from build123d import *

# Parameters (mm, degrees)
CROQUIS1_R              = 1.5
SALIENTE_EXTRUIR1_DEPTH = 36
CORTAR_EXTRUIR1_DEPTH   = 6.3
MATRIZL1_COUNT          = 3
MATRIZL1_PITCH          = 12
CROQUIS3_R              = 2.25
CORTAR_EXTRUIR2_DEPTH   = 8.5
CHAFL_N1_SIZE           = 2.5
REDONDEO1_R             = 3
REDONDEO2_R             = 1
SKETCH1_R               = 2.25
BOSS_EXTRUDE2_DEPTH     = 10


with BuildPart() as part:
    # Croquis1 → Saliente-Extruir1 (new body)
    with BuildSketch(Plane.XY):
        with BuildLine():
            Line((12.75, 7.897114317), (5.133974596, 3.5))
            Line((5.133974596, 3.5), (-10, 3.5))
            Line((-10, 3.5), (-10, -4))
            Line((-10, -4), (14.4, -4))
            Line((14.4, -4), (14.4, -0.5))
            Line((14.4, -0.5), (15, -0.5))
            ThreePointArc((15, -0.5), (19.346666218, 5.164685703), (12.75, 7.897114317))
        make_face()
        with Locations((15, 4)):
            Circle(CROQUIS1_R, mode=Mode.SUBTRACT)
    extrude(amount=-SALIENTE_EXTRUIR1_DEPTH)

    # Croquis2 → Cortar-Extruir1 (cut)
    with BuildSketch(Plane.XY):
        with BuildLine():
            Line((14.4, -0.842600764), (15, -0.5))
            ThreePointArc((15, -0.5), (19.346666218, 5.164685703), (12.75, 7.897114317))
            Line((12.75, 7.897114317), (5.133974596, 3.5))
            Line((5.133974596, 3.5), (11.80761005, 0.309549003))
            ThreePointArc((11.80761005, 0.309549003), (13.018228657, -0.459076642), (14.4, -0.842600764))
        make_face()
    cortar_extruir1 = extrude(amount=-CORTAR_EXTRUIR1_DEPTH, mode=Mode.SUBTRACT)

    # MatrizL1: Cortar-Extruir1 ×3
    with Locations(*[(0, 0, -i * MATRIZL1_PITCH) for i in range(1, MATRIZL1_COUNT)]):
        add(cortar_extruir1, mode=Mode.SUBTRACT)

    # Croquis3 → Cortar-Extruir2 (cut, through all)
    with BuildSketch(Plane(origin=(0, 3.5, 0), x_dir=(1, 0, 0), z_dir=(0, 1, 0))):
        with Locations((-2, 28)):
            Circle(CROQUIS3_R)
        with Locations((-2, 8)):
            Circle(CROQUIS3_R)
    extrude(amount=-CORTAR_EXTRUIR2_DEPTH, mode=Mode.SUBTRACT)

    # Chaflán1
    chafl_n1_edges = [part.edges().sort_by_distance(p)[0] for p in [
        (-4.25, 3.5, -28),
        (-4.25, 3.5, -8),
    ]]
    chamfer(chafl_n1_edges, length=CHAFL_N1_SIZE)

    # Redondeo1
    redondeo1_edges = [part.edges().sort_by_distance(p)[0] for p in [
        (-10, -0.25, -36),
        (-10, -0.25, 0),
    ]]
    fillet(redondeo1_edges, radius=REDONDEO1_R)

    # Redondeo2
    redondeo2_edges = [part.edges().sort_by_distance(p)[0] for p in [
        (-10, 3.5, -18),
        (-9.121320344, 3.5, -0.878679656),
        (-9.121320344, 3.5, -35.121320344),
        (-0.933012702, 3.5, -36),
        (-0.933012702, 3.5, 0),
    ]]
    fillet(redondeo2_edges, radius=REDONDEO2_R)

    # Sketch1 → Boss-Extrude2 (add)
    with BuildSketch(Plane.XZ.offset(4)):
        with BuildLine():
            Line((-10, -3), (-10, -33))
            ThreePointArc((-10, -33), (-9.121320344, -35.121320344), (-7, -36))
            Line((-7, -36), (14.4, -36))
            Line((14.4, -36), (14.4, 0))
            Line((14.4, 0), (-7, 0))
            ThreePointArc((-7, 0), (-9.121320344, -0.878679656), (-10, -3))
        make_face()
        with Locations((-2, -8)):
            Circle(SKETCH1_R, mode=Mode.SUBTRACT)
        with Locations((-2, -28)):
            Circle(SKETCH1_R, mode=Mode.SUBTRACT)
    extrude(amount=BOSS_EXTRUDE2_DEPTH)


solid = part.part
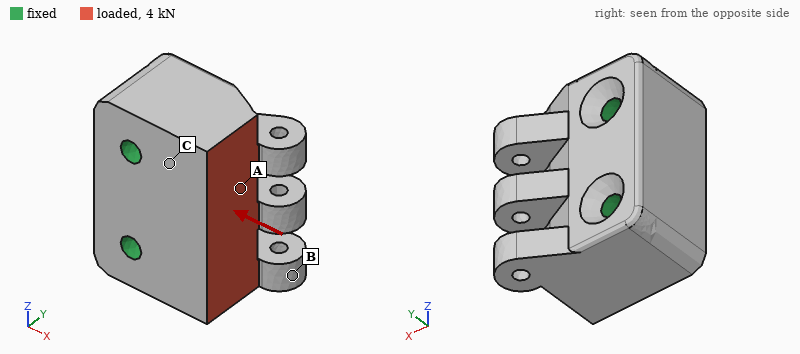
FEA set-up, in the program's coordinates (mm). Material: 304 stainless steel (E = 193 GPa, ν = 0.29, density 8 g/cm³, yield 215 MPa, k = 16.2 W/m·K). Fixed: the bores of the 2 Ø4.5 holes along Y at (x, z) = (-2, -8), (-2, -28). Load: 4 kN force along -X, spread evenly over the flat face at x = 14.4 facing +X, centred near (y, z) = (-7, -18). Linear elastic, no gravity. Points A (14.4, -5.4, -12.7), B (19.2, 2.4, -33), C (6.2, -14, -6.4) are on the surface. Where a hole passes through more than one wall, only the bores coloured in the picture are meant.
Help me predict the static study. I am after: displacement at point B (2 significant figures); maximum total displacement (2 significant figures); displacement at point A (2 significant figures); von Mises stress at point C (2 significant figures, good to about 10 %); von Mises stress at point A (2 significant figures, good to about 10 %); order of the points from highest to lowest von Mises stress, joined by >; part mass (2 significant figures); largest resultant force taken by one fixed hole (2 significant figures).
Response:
0.67 µm
1.1 µm
0.77 µm
11 MPa
7.0 MPa
C > A > B
120 g
2.0 kN
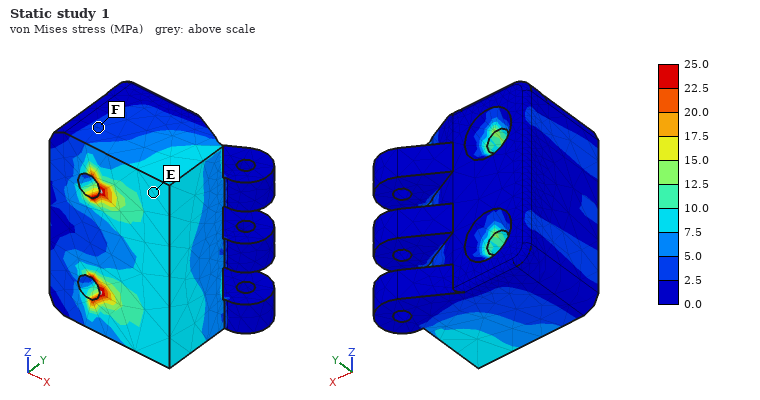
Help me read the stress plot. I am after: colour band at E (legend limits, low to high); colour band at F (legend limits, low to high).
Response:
7.5 to 10.0 MPa
2.5 to 5.0 MPa
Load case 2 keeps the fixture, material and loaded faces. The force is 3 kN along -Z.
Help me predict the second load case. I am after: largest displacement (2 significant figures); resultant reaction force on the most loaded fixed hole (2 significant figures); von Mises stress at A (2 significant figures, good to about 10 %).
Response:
2.9 µm
2.5 kN
13 MPa
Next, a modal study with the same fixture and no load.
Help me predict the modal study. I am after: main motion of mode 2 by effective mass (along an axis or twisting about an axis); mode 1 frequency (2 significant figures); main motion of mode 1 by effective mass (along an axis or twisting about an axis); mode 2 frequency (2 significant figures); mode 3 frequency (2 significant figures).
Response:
along Z
23 kHz
along Y
26 kHz
30 kHz
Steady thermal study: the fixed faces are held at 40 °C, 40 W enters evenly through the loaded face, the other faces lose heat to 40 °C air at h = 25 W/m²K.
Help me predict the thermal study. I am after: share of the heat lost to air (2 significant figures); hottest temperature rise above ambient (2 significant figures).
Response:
6.5 %
74 K
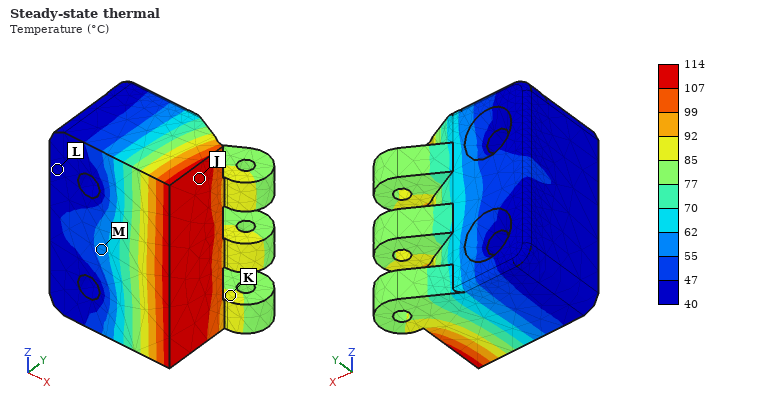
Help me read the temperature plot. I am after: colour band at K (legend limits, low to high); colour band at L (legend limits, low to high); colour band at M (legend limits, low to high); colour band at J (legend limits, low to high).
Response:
85 to 92 °C
40 to 47 °C
55 to 62 °C
107 to 114 °C
